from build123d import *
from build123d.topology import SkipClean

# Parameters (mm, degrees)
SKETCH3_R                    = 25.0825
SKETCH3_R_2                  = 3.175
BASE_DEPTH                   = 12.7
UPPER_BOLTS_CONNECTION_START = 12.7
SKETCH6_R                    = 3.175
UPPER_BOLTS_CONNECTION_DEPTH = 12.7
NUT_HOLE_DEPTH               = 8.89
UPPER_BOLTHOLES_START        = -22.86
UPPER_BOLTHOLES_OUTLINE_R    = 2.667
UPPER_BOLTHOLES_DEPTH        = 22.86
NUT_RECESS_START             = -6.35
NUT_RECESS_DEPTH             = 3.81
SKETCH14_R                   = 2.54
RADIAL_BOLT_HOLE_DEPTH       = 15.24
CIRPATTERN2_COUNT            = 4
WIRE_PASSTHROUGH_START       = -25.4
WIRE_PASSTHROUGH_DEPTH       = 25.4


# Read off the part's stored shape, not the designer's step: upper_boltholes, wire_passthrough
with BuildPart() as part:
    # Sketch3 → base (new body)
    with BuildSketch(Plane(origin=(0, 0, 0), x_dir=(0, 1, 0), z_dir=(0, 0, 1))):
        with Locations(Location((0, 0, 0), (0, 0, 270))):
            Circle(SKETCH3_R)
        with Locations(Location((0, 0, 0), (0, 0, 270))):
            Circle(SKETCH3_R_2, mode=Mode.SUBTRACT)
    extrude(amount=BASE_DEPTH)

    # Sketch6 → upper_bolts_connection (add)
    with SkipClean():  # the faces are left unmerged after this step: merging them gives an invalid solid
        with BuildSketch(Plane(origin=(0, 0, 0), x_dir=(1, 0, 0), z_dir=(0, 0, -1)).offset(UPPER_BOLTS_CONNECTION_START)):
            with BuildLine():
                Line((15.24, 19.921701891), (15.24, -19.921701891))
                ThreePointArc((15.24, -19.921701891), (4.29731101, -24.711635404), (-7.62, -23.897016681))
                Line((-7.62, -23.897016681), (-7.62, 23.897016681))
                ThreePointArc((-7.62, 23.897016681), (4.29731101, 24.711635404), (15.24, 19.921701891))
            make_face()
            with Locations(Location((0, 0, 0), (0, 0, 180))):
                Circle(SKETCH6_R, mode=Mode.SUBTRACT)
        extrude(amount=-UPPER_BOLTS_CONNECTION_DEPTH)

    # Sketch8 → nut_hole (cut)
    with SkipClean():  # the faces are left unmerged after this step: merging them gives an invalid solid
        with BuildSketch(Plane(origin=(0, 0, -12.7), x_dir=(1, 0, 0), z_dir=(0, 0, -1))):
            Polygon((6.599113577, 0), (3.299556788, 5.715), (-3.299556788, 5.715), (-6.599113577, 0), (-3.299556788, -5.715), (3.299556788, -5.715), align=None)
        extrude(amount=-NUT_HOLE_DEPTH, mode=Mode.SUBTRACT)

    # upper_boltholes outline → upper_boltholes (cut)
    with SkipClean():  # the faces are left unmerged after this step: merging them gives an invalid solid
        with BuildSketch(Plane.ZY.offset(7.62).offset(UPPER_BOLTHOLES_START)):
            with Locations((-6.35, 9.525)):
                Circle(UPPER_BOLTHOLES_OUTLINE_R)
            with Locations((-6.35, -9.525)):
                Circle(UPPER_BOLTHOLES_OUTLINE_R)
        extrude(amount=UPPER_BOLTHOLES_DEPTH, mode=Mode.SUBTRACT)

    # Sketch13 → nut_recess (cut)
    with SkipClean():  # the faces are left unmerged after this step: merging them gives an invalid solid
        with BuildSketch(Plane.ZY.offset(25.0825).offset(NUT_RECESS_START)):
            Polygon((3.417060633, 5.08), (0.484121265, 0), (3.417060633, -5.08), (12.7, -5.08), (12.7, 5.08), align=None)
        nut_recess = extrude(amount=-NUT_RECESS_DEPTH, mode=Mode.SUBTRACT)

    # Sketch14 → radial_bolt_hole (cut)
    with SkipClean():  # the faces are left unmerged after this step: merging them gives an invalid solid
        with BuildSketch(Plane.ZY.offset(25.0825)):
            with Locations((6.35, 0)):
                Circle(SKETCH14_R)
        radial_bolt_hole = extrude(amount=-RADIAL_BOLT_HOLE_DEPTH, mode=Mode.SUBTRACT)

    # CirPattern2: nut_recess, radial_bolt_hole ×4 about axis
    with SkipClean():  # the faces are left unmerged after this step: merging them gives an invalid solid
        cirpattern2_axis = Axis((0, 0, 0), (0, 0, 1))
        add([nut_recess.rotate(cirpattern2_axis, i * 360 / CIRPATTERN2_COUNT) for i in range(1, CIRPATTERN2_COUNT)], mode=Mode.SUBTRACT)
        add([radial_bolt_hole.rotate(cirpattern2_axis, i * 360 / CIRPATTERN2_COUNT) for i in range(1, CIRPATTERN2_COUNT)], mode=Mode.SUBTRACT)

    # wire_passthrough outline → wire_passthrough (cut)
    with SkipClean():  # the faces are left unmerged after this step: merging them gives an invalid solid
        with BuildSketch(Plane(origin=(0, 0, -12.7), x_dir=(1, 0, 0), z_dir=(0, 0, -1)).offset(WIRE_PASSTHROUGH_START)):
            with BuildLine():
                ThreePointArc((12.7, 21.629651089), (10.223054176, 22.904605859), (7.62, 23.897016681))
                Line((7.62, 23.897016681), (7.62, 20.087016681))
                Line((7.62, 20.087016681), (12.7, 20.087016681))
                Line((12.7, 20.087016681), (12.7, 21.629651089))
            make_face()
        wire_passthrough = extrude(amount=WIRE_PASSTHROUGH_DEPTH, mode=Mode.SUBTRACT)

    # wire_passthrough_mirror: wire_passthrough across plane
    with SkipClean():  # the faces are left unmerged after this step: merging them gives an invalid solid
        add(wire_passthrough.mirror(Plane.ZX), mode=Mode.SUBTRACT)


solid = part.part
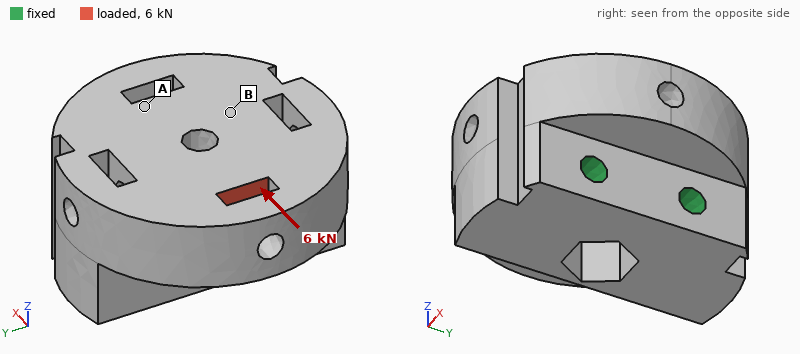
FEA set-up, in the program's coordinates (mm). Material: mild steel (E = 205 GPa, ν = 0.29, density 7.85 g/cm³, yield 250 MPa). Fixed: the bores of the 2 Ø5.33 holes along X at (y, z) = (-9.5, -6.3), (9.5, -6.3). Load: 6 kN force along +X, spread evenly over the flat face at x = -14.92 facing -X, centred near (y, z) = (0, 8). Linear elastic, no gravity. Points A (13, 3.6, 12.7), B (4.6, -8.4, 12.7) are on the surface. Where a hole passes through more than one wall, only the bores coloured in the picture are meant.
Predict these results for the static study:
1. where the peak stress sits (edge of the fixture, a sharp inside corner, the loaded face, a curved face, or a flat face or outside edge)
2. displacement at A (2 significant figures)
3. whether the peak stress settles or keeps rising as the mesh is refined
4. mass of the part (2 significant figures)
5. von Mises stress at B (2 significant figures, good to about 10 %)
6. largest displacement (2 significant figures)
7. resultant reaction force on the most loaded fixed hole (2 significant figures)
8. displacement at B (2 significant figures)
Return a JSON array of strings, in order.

["edge of the fixture", "2.6 µm", "keeps rising", "260 g", "13 MPa", "8.2 µm", "3.0 kN", "2.8 µm"]
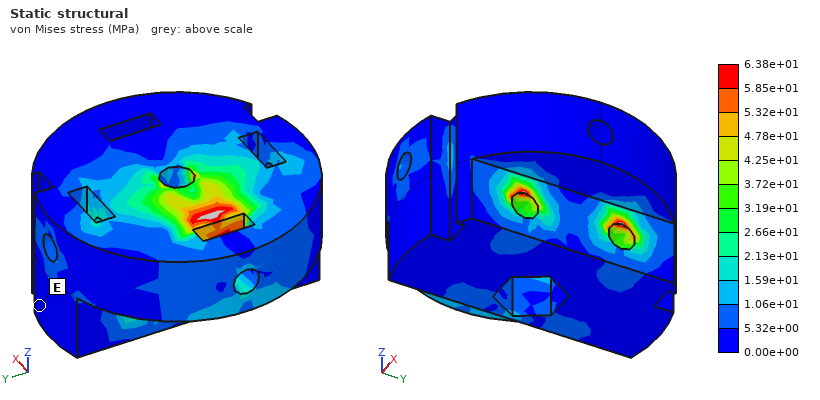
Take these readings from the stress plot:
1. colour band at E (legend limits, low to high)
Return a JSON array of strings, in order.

["0.00e+00 to 5.32e+00 MPa"]
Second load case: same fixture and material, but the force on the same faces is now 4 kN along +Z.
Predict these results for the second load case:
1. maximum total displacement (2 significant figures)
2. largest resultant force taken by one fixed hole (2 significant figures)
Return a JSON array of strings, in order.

["12 µm", "2.1 kN"]
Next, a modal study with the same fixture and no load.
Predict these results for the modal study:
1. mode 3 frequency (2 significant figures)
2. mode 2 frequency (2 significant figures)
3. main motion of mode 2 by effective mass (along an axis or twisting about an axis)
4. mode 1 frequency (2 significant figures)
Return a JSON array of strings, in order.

["21 kHz", "18 kHz", "along Y", "15 kHz"]
